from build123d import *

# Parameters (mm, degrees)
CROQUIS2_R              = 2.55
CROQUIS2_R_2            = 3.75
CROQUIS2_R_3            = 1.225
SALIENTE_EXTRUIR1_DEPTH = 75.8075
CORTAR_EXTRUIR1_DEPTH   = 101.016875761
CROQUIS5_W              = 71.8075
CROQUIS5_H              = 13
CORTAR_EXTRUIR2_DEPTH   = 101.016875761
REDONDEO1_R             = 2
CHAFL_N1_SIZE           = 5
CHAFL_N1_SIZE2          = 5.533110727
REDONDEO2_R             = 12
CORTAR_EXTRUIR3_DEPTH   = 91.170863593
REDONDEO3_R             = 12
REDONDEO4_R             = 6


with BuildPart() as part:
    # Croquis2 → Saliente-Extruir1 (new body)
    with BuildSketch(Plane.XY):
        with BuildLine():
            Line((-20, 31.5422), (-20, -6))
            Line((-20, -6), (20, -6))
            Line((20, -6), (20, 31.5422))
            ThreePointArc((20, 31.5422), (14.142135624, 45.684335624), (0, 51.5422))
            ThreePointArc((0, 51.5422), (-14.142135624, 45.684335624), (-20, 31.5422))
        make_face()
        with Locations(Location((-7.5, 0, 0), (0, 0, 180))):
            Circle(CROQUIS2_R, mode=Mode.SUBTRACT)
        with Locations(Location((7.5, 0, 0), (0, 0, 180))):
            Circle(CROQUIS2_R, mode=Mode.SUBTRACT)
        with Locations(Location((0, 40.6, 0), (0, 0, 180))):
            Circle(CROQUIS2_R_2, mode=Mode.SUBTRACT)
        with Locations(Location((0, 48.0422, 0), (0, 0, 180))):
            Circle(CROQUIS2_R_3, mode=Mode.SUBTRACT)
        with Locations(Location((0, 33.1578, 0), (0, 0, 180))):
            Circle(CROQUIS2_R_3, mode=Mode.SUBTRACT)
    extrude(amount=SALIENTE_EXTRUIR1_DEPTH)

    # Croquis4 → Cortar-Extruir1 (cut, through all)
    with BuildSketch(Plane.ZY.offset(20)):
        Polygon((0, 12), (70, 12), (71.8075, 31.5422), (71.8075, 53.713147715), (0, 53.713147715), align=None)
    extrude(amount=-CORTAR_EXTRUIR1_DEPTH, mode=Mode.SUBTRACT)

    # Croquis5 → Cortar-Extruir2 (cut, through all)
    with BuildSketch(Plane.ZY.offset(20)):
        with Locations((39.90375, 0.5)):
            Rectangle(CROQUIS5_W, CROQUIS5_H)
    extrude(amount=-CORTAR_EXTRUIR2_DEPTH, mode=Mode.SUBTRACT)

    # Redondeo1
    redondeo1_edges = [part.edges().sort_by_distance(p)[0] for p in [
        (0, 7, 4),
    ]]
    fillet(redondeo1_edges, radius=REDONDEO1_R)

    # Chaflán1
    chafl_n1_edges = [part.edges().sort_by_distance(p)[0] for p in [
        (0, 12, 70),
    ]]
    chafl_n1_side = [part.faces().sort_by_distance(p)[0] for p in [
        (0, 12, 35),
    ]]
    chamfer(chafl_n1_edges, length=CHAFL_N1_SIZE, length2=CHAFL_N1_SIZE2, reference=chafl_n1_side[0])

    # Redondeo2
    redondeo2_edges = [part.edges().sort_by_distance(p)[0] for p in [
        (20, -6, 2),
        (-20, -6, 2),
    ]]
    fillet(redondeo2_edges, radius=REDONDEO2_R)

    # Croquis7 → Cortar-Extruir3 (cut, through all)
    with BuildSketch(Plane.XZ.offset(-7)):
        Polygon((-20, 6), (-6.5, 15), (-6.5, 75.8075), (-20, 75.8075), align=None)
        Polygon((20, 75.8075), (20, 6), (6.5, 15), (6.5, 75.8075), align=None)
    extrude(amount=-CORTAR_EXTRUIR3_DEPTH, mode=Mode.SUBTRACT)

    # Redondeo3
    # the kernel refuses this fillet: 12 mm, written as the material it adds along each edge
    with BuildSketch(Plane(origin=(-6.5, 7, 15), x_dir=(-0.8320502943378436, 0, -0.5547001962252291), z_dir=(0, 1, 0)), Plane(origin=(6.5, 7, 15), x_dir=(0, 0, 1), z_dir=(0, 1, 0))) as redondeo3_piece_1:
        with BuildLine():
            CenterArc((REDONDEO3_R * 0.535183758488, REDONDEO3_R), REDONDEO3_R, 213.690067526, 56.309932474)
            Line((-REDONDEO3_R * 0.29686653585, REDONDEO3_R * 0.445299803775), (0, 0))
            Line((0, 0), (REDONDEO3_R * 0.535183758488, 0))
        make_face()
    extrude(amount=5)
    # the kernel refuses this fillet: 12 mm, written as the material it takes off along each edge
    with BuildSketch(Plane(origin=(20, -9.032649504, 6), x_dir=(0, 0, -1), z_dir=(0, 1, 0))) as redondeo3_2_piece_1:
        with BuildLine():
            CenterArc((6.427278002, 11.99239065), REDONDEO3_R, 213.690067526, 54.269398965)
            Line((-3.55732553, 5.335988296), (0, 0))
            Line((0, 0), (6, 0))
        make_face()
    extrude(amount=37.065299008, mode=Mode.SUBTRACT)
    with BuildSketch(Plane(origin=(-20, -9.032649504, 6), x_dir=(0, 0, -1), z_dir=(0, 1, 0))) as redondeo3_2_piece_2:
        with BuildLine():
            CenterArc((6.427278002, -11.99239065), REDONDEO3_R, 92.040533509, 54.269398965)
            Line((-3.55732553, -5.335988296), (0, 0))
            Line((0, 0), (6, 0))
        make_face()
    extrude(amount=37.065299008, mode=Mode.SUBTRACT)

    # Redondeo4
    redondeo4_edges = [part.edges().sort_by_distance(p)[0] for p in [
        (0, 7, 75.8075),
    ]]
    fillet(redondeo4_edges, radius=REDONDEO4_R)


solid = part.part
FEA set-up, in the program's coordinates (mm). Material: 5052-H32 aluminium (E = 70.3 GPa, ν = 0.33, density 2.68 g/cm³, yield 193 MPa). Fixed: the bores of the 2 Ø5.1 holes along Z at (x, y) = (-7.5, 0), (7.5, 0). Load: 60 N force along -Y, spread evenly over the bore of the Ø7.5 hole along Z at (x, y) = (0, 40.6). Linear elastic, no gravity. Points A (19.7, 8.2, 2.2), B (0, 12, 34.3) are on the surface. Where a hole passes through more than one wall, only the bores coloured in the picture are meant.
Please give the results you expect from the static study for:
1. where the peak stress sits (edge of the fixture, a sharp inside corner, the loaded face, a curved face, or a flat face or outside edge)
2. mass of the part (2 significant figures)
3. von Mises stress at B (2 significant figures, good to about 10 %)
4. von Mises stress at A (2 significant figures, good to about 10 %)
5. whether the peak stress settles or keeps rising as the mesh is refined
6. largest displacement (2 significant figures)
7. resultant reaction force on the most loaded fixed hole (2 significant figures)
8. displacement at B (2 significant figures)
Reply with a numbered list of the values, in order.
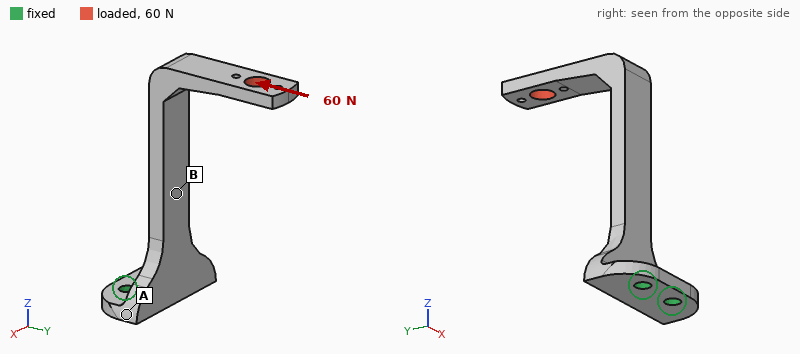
1. edge of the fixture
2. 27 g
3. 44 MPa
4. 11 MPa
5. keeps rising
6. 1.0 mm
7. 48 N
8. 0.20 mm
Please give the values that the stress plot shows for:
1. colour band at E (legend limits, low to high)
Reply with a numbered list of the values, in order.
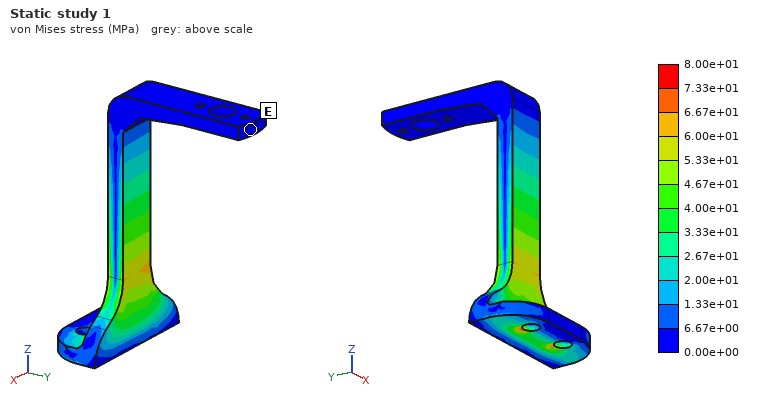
1. 0.00e+00 to 6.67e+00 MPa
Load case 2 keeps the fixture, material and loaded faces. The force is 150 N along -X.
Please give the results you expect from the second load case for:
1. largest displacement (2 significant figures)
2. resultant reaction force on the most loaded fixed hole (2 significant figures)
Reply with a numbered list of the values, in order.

1. 1.2 mm
2. 640 N
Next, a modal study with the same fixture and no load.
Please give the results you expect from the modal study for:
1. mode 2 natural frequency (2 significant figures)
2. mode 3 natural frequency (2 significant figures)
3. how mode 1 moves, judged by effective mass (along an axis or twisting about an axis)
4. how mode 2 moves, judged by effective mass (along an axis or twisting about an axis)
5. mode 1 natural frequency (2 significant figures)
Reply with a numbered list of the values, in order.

1. 1000 Hz
2. 1900 Hz
3. along Y
4. along X
5. 450 Hz
